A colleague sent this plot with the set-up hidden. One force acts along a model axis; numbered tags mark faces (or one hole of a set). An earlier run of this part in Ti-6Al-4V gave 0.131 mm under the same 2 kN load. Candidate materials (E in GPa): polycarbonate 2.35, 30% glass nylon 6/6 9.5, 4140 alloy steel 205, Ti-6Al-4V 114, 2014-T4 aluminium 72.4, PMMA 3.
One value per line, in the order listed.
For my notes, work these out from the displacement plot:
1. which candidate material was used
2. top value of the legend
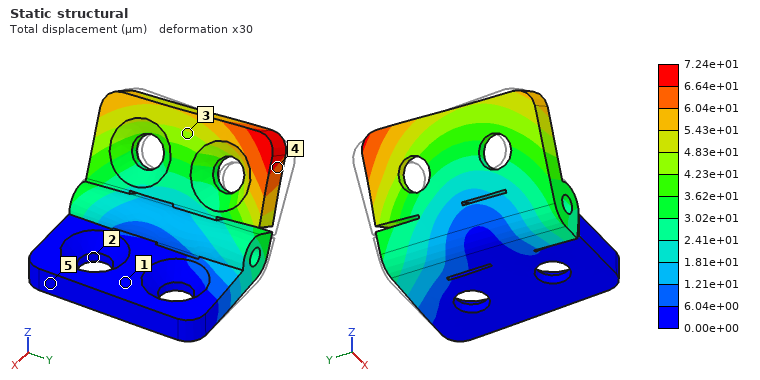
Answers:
4140 alloy steel
7.24e+01 µm
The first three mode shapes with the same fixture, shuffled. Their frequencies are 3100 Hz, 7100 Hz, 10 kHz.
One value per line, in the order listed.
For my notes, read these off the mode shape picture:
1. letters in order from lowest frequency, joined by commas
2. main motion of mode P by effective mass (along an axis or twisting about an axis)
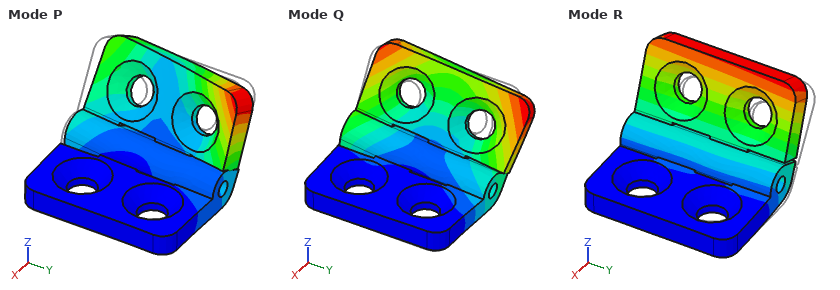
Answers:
R, Q, P
along Y
